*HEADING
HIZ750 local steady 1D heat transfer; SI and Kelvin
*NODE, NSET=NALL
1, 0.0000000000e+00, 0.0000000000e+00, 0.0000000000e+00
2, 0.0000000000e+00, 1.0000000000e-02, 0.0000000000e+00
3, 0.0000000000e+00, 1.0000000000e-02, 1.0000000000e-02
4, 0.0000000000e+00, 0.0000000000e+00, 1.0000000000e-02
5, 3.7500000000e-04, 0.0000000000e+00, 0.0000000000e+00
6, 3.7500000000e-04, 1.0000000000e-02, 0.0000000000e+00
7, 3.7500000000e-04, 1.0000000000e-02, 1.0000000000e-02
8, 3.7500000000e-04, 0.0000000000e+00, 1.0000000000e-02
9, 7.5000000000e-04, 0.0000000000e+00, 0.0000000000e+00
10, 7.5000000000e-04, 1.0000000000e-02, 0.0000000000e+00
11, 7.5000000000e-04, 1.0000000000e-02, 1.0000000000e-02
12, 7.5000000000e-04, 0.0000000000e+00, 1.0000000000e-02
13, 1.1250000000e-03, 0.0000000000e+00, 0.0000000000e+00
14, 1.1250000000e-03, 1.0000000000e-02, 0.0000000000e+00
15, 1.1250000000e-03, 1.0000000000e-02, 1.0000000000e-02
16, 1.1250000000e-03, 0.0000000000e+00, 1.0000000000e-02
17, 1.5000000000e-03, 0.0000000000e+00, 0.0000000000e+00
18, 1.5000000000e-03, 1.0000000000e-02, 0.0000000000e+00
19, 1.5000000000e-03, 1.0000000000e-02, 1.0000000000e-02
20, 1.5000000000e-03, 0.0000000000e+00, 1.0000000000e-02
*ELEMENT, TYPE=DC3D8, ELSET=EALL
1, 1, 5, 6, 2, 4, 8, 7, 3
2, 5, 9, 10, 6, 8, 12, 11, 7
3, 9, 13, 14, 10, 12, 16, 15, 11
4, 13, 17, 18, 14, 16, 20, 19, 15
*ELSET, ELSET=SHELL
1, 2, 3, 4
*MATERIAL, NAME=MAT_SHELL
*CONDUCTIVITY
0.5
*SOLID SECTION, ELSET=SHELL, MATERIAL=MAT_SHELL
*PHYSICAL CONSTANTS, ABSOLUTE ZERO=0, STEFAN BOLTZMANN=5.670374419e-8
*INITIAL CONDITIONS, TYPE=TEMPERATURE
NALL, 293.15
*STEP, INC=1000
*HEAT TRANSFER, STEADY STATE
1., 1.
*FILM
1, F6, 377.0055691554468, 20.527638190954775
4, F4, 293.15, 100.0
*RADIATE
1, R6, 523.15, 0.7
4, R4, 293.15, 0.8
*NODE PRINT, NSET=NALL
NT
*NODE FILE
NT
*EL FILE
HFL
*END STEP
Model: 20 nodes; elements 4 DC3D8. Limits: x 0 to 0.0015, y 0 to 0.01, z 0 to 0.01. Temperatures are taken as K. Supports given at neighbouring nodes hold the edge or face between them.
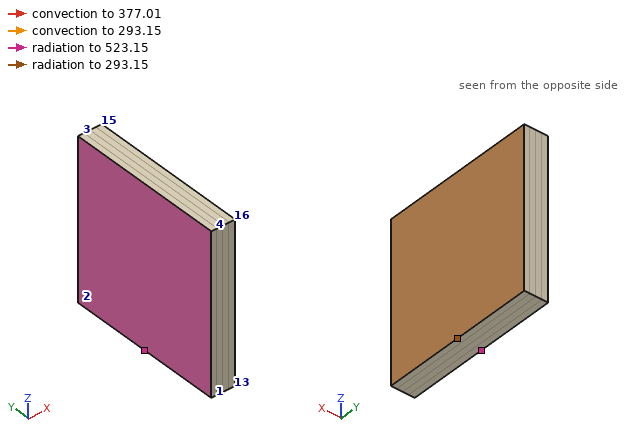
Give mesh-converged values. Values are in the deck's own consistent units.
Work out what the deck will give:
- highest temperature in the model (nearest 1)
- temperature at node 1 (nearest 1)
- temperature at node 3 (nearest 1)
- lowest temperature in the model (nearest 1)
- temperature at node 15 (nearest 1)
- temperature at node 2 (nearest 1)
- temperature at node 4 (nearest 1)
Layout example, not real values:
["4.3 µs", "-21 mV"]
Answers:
["335 K", "335 K", "335 K", "325 K", "327 K", "335 K", "335 K"]
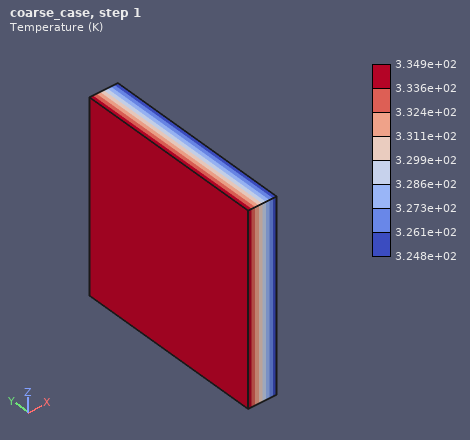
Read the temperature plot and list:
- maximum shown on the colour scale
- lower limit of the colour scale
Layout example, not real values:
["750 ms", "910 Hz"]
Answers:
["3.349e+02 K", "3.248e+02 K"]
